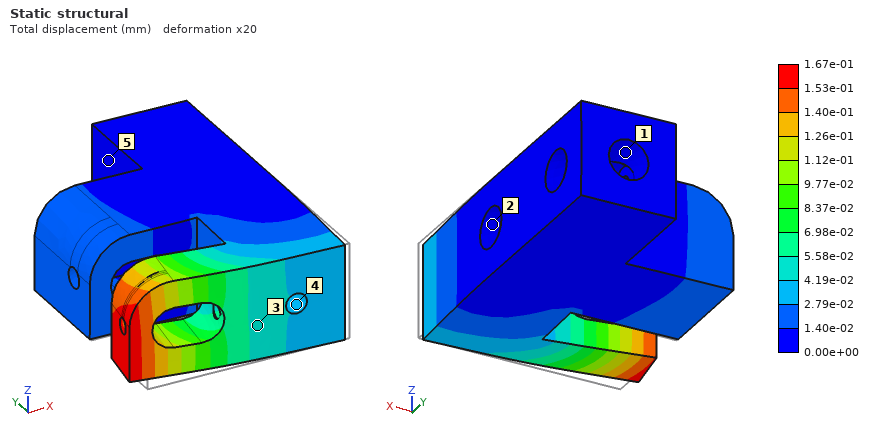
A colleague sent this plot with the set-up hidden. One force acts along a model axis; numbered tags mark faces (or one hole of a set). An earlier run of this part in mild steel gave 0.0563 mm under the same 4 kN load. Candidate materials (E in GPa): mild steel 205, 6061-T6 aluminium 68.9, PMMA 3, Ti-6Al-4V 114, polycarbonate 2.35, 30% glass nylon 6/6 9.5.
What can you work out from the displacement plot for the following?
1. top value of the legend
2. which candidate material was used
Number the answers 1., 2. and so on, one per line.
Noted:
1. 1.67e-01 mm
2. 6061-T6 aluminium
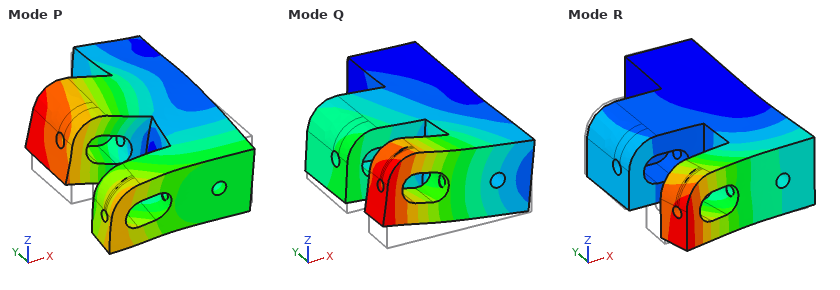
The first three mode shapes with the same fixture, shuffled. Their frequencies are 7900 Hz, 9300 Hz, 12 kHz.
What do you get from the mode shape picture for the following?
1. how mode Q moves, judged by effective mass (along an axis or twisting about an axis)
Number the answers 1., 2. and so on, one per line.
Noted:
1. along Z
